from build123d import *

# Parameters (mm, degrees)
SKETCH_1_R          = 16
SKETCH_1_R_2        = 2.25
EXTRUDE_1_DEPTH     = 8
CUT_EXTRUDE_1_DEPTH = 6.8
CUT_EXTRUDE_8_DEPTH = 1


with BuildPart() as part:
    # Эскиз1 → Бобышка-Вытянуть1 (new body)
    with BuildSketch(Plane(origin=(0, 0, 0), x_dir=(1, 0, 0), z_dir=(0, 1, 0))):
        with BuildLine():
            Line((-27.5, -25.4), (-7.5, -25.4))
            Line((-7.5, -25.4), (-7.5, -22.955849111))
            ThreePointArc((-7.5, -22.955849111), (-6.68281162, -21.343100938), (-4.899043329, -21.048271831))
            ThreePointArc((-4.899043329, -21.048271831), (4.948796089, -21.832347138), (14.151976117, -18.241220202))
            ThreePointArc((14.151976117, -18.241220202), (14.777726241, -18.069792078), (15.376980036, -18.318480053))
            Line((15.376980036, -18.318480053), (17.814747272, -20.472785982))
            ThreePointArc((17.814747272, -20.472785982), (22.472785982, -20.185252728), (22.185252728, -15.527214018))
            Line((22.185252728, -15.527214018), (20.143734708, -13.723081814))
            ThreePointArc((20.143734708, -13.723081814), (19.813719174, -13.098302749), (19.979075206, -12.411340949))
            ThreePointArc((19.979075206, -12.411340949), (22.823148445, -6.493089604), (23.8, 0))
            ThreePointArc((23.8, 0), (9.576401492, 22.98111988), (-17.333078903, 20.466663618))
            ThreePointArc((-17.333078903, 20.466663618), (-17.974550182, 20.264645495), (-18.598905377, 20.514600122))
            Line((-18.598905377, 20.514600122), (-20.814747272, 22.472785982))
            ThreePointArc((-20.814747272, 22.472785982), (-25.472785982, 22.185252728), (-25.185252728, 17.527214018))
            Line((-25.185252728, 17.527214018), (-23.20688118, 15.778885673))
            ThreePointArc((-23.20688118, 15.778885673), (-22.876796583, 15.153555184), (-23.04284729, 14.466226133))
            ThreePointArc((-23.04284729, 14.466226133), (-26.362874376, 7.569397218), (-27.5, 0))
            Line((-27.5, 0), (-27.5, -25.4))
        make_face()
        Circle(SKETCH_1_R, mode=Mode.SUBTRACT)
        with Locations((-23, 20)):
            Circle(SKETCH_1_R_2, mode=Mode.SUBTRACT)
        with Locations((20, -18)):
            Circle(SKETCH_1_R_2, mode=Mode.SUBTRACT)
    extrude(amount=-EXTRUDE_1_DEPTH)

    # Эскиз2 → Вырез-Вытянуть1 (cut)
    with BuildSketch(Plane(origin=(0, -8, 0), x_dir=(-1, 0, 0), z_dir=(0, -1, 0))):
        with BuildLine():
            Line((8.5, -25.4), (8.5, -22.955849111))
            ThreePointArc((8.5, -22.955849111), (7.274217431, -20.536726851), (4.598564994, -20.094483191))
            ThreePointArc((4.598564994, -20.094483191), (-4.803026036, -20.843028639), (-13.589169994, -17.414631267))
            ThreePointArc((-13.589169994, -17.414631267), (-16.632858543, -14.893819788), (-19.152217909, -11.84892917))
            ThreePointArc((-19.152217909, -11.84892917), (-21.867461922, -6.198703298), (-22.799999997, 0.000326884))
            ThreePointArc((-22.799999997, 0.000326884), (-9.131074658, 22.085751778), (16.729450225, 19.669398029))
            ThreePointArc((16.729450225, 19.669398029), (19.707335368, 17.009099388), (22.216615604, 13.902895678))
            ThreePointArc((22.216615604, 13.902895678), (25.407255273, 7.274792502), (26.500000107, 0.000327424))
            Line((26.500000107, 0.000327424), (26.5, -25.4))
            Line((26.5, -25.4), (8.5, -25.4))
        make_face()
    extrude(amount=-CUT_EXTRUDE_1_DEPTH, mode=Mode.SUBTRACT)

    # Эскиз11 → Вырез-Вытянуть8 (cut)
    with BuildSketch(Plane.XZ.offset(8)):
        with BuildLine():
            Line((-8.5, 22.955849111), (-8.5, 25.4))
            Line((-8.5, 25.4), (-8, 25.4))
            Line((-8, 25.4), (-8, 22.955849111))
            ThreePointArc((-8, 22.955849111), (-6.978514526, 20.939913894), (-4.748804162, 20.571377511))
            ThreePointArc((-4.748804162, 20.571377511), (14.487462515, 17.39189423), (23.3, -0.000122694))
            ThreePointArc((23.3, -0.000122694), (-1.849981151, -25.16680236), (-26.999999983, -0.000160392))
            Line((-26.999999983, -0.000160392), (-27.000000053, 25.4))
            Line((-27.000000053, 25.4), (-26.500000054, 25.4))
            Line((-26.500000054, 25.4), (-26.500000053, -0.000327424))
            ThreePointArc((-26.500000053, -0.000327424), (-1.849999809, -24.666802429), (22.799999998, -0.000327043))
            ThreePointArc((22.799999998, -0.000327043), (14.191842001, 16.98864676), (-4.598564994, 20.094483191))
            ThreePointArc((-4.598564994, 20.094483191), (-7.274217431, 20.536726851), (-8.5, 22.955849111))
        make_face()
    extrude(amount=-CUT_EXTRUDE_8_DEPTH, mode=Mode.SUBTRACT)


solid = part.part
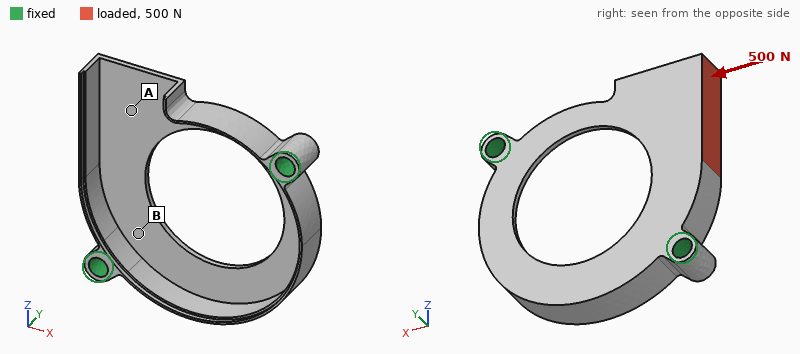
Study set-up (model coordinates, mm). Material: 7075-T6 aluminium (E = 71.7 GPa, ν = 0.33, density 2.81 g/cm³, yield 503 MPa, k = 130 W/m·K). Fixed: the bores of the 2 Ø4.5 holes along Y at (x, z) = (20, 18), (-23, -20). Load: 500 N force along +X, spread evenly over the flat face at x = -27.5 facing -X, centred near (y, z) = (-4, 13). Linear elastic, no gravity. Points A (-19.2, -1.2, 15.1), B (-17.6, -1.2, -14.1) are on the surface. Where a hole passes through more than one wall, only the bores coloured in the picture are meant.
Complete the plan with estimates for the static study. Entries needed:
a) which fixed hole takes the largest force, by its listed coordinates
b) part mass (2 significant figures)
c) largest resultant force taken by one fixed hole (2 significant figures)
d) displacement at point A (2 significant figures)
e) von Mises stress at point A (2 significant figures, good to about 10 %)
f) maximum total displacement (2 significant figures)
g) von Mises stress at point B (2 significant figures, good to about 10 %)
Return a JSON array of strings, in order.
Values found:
["(20, 18)", "8.3 g", "390 N", "0.15 mm", "150 MPa", "0.55 mm", "45 MPa"]
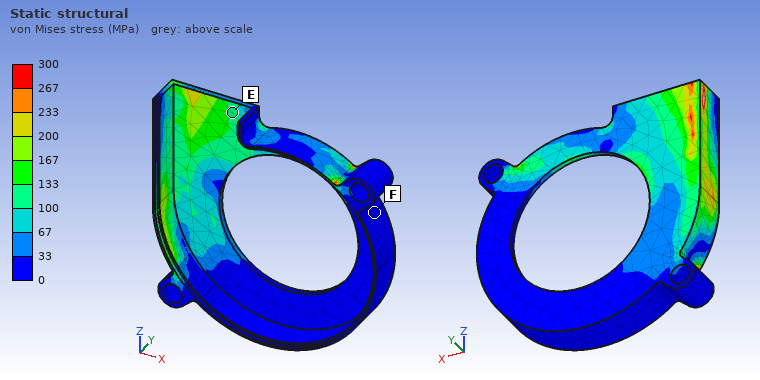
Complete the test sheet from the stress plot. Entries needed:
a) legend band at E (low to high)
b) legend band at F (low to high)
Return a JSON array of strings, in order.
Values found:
["100 to 133 MPa", "0 to 33 MPa"]
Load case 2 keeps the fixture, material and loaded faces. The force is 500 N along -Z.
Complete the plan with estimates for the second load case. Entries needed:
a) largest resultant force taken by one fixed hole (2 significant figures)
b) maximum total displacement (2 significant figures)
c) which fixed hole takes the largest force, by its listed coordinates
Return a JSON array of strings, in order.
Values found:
["510 N", "0.27 mm", "(-23, -20)"]
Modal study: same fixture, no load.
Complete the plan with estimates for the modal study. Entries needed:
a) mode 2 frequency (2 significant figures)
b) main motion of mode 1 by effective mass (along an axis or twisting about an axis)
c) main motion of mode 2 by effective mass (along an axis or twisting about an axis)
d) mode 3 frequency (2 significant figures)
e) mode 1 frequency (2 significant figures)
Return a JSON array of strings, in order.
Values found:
["4000 Hz", "along Y", "along Y", "4800 Hz", "2400 Hz"]
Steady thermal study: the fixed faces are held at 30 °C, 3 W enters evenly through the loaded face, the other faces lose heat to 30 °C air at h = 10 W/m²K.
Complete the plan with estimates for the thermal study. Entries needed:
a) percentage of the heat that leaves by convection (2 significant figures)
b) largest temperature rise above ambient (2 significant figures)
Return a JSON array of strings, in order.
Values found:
["10 %", "24 K"]
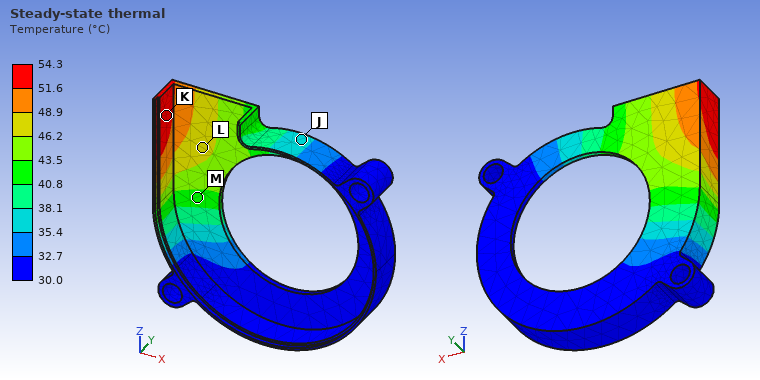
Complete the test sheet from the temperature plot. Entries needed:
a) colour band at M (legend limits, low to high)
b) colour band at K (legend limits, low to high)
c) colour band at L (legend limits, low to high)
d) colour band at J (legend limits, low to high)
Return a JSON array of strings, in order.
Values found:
["40.8 to 43.5 °C", "51.6 to 54.3 °C", "46.2 to 48.9 °C", "35.4 to 38.1 °C"]
